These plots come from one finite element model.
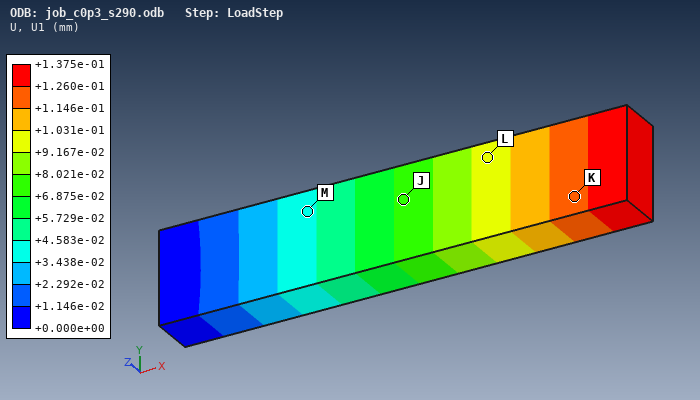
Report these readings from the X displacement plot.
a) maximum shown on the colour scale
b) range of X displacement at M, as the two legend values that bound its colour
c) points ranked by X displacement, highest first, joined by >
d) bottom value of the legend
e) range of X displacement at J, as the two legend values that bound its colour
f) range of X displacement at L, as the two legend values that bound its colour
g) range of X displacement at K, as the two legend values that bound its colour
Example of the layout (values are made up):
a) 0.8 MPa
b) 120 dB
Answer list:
a) +1.375e-01 mm
b) +3.438e-02 to +4.583e-02 mm
c) K > L > J > M
d) +0.000e+00 mm
e) +6.875e-02 to +8.021e-02 mm
f) +9.167e-02 to +1.031e-01 mm
g) +1.146e-01 to +1.260e-01 mm
